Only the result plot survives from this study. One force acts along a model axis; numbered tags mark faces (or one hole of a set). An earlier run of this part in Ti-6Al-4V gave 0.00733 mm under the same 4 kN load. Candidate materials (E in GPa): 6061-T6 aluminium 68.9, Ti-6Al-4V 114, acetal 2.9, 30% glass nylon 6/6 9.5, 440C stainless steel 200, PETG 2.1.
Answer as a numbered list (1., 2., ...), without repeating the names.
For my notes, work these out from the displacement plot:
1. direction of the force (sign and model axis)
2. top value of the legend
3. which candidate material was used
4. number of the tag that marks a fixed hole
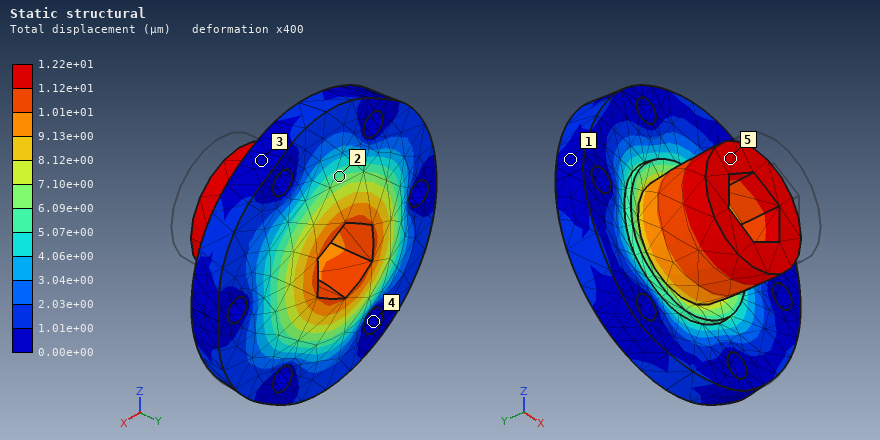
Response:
1. +Y
2. 1.22e+01 µm
3. 6061-T6 aluminium
4. 4
